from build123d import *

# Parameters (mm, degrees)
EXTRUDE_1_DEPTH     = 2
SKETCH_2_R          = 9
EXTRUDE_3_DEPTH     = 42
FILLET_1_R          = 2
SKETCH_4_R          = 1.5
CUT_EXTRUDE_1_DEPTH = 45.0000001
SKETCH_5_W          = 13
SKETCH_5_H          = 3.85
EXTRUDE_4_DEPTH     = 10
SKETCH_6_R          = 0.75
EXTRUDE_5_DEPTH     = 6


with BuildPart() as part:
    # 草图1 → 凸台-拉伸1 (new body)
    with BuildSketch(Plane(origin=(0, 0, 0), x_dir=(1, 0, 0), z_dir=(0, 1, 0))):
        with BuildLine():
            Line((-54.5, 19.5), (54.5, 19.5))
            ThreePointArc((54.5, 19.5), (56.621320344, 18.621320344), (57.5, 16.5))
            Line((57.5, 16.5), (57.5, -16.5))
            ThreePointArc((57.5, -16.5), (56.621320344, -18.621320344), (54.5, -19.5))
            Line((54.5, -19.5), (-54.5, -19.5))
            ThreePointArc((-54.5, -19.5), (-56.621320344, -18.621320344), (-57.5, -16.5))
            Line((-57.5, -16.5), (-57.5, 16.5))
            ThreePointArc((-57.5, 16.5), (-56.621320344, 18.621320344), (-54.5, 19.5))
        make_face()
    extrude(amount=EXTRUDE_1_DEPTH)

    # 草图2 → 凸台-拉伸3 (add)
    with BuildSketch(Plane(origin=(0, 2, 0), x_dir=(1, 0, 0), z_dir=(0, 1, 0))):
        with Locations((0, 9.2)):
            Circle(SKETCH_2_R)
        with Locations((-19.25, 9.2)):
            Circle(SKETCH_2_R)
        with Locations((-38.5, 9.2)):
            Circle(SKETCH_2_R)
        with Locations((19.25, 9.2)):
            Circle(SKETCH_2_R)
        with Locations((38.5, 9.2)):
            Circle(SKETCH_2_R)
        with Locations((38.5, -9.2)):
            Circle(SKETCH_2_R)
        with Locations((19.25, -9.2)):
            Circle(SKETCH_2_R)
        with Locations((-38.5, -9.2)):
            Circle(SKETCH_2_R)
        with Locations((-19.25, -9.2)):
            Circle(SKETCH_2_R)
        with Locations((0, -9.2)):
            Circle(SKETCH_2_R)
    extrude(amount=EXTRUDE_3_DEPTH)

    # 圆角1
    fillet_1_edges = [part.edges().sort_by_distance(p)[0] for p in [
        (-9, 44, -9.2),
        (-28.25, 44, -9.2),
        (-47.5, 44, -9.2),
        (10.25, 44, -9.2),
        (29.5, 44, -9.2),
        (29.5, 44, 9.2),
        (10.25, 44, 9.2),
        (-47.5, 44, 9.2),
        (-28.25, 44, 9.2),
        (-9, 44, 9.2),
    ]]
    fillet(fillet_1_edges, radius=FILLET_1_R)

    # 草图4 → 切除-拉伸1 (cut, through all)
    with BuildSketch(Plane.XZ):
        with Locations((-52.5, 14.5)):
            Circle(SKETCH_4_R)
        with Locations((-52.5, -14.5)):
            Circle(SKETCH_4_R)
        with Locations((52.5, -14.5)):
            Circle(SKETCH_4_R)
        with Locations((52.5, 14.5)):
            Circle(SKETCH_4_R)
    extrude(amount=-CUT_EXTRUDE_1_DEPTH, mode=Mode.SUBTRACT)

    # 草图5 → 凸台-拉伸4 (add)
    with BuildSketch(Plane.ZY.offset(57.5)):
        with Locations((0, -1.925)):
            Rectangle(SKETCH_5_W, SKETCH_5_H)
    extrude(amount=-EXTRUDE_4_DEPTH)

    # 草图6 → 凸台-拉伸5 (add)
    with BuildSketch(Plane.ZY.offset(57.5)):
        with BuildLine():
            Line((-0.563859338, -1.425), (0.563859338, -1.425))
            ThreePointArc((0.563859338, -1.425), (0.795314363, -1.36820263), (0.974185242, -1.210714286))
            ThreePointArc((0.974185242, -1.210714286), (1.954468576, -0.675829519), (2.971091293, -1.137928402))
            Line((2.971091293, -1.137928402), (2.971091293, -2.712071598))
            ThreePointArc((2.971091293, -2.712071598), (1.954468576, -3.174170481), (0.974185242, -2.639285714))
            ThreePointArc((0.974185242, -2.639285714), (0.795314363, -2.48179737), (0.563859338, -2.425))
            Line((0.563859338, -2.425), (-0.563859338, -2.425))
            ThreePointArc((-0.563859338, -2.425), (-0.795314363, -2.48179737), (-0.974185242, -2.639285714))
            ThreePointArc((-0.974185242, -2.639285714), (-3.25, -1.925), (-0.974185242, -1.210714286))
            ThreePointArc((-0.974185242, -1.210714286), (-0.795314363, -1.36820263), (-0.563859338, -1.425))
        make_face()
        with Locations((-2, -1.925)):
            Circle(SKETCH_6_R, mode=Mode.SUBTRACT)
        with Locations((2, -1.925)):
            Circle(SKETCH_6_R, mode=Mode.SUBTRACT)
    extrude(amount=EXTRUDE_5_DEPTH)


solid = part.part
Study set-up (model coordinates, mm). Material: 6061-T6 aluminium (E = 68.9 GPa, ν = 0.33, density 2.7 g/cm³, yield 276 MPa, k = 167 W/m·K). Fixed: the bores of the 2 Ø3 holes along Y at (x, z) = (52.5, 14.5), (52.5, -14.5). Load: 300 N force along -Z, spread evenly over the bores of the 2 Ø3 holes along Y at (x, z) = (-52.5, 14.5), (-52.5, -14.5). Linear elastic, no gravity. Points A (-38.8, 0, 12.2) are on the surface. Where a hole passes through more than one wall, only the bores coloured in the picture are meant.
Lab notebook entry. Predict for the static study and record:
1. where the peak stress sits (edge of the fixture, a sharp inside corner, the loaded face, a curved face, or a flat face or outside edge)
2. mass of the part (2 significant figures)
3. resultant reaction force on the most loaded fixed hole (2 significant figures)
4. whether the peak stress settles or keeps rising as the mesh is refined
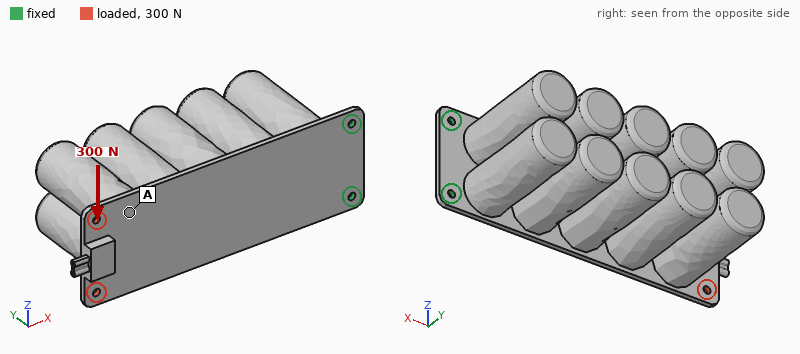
edge of the fixture
310 g
1.1 kN
keeps rising
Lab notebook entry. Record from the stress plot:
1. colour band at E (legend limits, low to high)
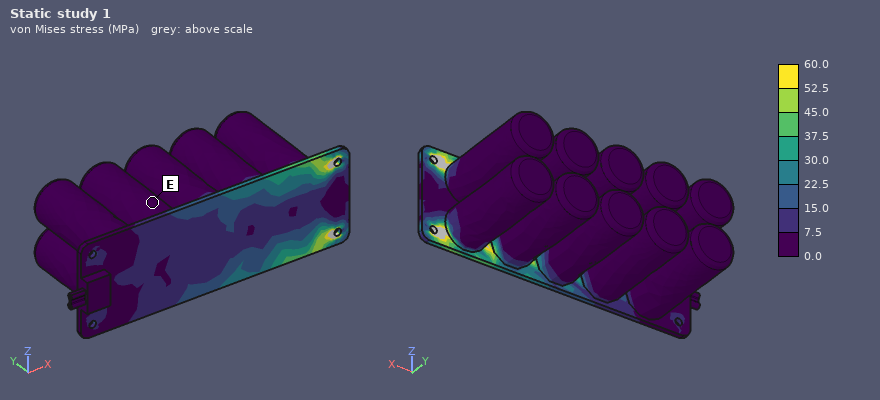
0.0 to 7.5 MPa
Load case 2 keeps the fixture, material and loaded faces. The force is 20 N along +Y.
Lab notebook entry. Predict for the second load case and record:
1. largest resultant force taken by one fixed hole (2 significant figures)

11 N
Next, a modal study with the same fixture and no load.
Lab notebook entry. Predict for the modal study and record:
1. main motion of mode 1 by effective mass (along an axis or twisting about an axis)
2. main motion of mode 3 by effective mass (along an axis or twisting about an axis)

along Y
along Z
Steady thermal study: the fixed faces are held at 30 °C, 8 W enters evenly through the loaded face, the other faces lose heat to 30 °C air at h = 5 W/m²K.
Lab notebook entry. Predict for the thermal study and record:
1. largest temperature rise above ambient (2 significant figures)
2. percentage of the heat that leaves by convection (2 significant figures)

34 K
31 %
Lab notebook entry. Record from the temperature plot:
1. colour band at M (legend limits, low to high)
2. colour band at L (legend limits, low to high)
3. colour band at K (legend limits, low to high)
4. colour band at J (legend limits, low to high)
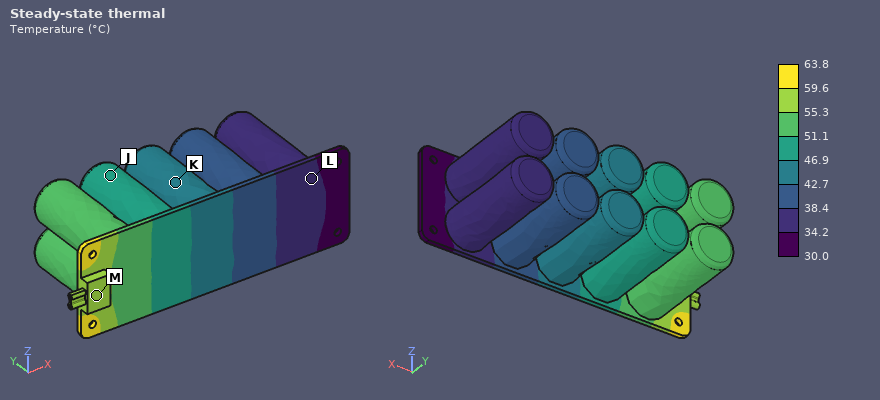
55.3 to 59.6 °C
34.2 to 38.4 °C
42.7 to 46.9 °C
46.9 to 51.1 °C
